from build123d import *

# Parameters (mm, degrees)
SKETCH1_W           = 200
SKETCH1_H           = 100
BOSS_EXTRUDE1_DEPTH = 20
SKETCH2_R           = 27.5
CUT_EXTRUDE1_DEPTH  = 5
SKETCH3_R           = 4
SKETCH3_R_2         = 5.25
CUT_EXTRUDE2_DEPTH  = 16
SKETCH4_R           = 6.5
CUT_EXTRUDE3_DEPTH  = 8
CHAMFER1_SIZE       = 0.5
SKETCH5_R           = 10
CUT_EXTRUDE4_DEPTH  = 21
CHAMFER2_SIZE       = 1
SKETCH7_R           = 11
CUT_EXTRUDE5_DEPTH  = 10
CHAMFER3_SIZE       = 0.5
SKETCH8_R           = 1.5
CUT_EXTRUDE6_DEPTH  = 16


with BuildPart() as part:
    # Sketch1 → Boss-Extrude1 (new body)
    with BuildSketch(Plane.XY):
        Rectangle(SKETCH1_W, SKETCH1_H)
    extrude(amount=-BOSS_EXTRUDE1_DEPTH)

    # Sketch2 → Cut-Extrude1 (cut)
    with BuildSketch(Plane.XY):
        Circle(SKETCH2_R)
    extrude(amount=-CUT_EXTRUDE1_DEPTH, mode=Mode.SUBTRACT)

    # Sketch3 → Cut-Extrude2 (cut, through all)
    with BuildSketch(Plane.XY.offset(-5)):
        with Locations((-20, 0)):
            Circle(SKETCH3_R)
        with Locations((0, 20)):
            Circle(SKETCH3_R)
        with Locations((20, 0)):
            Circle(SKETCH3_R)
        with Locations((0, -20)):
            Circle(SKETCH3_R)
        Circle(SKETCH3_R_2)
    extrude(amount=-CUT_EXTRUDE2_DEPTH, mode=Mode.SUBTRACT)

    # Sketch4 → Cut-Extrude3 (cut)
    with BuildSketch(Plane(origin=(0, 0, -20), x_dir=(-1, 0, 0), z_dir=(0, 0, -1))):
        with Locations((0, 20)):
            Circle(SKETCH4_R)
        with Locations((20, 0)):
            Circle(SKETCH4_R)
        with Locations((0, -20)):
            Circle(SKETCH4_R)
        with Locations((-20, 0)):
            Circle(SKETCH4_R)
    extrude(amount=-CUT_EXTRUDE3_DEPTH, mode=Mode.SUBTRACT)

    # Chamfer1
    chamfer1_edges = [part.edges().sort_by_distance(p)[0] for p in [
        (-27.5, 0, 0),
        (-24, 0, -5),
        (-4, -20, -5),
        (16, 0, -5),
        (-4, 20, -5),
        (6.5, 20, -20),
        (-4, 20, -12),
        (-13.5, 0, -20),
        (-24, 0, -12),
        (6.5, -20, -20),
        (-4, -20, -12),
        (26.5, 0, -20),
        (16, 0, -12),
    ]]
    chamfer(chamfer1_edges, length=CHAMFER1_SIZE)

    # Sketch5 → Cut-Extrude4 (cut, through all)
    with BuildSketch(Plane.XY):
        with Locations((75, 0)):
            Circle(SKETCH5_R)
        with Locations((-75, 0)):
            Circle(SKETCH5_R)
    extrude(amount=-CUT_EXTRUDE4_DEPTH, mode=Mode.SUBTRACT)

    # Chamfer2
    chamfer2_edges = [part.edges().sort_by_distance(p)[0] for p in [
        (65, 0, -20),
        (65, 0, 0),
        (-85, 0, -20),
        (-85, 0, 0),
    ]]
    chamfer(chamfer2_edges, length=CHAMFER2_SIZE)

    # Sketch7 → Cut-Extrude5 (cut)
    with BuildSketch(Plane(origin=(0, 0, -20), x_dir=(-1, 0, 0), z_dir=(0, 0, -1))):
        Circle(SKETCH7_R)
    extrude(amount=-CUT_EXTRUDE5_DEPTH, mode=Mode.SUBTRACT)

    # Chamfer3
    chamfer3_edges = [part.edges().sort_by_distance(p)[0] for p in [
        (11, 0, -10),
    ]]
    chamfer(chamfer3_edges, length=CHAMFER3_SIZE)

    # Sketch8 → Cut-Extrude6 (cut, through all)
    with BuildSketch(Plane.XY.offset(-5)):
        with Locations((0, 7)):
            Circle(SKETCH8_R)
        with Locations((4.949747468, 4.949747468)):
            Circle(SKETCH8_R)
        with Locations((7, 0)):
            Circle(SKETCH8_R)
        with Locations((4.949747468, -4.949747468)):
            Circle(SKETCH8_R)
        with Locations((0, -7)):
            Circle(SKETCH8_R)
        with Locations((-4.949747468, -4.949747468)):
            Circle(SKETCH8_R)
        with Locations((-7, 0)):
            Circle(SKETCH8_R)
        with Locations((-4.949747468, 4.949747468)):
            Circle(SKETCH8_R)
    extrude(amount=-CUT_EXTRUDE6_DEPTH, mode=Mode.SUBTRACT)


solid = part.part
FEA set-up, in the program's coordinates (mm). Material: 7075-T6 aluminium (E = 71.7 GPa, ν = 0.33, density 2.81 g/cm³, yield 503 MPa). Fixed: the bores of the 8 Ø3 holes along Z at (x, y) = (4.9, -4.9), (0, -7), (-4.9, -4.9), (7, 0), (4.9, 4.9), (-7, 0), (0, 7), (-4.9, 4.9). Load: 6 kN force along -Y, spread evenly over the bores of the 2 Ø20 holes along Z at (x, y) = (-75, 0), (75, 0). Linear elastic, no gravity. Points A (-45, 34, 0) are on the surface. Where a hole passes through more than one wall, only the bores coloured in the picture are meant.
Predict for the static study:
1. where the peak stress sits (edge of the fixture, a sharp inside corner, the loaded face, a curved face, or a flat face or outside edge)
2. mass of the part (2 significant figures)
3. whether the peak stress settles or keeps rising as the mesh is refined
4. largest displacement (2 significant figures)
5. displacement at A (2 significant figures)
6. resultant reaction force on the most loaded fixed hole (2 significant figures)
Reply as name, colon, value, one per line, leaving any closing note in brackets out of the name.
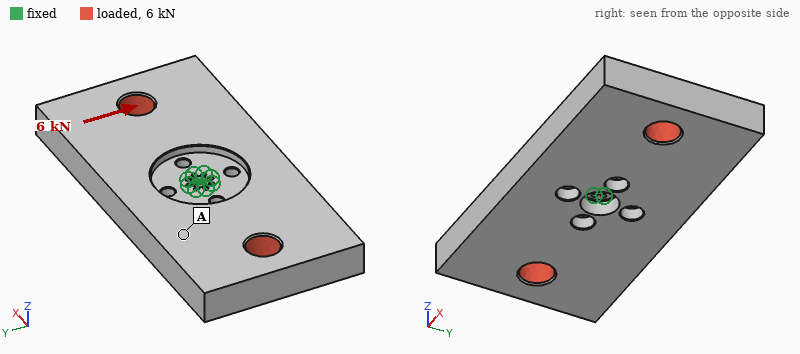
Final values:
where the peak stress sits: edge of the fixture
mass of the part: 1.0 kg
whether the peak stress settles or keeps rising as the mesh is refined: keeps rising
largest displacement: 31 µm
displacement at A: 17 µm
resultant reaction force on the most loaded fixed hole: 1000 N
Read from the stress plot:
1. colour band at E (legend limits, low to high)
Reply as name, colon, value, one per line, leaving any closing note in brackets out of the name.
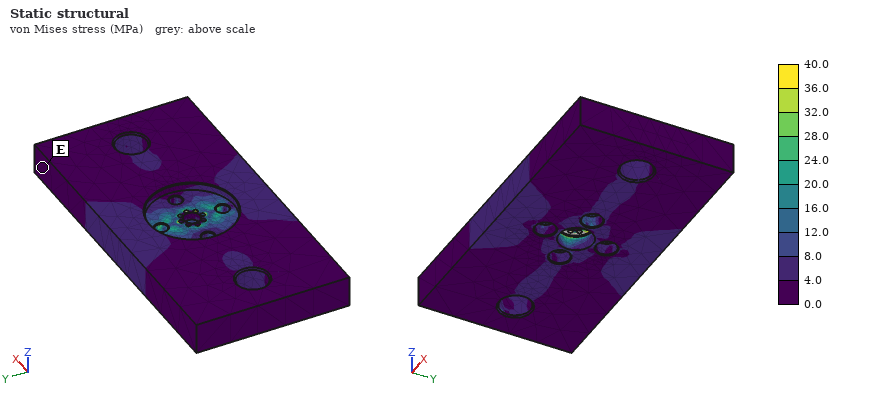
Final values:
colour band at E: 0.0 to 4.0 MPa
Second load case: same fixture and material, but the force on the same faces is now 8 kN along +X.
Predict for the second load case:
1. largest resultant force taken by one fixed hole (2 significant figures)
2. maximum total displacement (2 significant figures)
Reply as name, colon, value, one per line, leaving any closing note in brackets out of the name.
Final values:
largest resultant force taken by one fixed hole: 1.3 kN
maximum total displacement: 62 µm
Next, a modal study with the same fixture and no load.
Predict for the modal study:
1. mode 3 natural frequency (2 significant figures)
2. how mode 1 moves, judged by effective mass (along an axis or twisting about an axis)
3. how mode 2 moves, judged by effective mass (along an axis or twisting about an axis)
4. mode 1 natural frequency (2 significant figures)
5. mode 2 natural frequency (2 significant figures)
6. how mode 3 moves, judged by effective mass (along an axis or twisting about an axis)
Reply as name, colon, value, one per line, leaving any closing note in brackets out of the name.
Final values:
mode 3 natural frequency: 930 Hz
how mode 1 moves, judged by effective mass: twisting about Y
how mode 2 moves, judged by effective mass: twisting about Z
mode 1 natural frequency: 480 Hz
mode 2 natural frequency: 870 Hz
how mode 3 moves, judged by effective mass: twisting about X
